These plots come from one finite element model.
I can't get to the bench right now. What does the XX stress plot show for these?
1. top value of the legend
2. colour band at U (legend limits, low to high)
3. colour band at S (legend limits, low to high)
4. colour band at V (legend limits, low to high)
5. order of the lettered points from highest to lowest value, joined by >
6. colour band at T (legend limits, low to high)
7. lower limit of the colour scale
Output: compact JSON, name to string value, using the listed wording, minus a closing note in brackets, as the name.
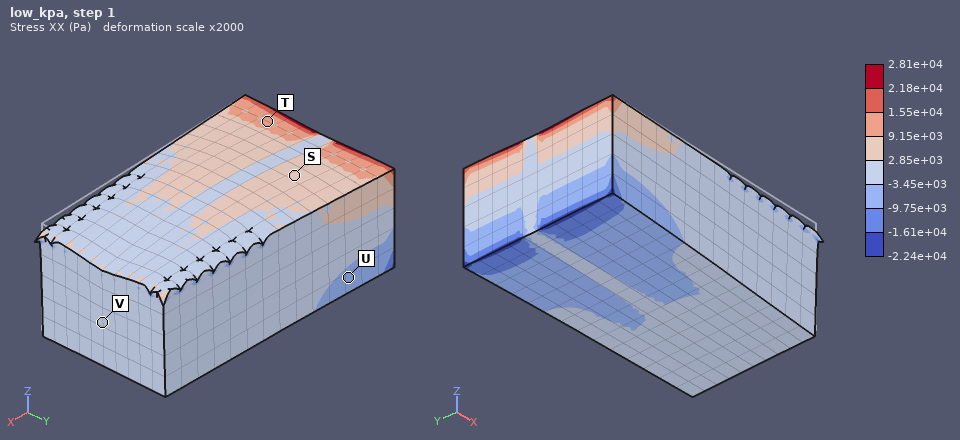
{"top value of the legend": "2.81e+04 Pa", "colour band at U": "-9.75e+03 to -3.45e+03 Pa", "colour band at S": "2.85e+03 to 9.15e+03 Pa", "colour band at V": "-3.45e+03 to 2.85e+03 Pa", "order of the lettered points from highest to lowest value, joined by >": "T > S > V > U", "colour band at T": "9.15e+03 to 1.55e+04 Pa", "lower limit of the colour scale": "-2.24e+04 Pa"}
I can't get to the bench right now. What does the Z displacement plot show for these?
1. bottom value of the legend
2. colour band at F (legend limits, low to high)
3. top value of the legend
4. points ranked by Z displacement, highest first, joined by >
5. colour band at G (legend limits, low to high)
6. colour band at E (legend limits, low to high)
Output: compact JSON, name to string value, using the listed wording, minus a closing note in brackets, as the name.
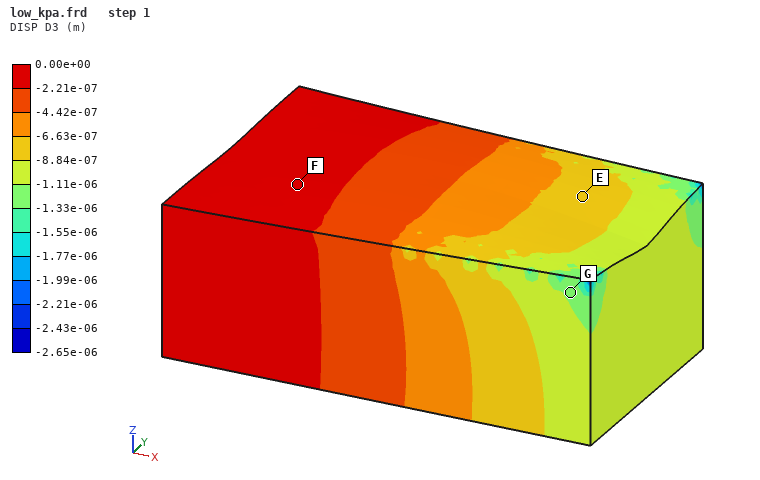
{"bottom value of the legend": "-2.65e-06 m", "colour band at F": "-2.21e-07 to 0.00e+00 m", "top value of the legend": "0.00e+00 m", "points ranked by Z displacement, highest first, joined by >": "F > E > G", "colour band at G": "-1.33e-06 to -1.11e-06 m", "colour band at E": "-8.84e-07 to -6.63e-07 m"}
